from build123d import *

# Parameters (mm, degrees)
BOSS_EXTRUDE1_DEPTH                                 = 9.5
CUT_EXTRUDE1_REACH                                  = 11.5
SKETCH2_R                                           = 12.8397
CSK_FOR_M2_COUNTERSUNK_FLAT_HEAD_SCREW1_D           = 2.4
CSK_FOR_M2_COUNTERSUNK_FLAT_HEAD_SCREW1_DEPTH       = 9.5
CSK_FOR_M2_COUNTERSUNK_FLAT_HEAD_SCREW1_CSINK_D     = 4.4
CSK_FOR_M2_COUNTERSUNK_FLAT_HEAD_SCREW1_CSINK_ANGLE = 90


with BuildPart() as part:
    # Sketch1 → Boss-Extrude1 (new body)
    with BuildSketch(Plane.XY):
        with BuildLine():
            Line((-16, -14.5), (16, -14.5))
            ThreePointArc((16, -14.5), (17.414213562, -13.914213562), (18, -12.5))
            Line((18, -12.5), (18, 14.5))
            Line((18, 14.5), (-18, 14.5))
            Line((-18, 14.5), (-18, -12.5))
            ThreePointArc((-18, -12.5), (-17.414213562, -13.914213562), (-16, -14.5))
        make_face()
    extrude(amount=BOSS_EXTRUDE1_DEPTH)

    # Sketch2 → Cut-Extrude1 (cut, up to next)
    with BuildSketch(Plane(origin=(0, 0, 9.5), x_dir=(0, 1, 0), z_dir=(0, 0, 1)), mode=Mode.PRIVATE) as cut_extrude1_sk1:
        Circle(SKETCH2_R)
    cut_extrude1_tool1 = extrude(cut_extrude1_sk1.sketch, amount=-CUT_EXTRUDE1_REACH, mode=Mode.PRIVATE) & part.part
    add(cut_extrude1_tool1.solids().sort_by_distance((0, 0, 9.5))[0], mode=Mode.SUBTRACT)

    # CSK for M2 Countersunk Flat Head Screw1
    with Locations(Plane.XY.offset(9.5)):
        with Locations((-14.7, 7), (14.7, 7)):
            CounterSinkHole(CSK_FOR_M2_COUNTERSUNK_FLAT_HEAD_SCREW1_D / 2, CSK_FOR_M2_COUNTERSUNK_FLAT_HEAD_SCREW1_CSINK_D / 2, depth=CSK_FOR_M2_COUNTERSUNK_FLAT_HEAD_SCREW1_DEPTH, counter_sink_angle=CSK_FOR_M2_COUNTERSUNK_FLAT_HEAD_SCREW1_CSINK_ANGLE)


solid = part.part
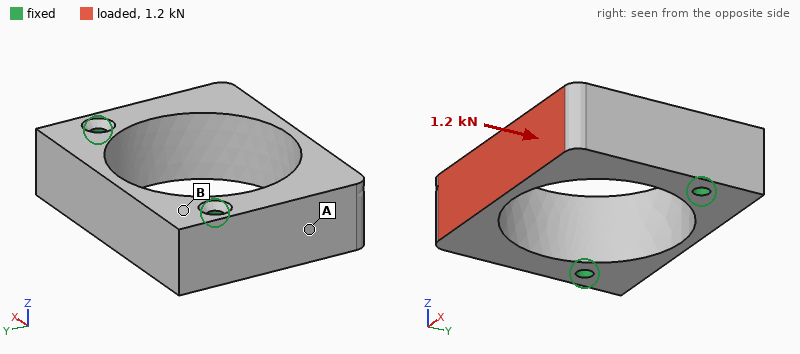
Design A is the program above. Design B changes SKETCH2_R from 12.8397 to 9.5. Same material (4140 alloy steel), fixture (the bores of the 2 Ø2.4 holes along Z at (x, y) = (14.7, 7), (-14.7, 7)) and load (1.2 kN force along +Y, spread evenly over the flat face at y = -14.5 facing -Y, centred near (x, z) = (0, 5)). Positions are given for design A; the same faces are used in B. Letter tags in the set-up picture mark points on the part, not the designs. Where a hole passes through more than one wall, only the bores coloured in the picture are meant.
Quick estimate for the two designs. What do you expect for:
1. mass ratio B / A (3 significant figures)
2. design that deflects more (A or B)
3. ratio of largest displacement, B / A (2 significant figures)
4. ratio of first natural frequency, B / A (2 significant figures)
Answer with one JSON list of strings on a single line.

["1.46", "A", "0.22", "1.1"]
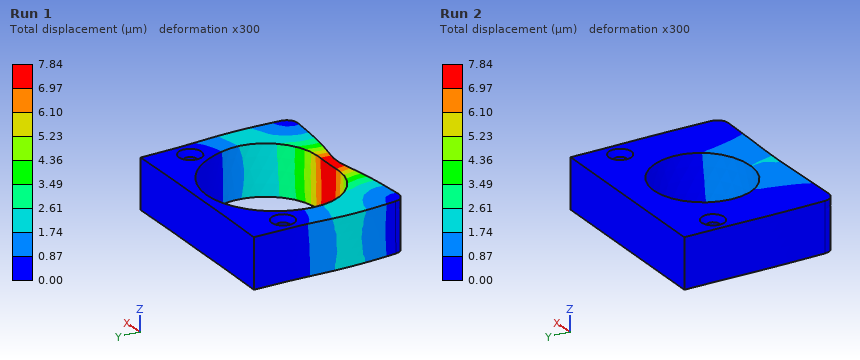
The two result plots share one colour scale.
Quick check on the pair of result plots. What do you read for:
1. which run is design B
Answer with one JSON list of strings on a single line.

["Run 2"]
